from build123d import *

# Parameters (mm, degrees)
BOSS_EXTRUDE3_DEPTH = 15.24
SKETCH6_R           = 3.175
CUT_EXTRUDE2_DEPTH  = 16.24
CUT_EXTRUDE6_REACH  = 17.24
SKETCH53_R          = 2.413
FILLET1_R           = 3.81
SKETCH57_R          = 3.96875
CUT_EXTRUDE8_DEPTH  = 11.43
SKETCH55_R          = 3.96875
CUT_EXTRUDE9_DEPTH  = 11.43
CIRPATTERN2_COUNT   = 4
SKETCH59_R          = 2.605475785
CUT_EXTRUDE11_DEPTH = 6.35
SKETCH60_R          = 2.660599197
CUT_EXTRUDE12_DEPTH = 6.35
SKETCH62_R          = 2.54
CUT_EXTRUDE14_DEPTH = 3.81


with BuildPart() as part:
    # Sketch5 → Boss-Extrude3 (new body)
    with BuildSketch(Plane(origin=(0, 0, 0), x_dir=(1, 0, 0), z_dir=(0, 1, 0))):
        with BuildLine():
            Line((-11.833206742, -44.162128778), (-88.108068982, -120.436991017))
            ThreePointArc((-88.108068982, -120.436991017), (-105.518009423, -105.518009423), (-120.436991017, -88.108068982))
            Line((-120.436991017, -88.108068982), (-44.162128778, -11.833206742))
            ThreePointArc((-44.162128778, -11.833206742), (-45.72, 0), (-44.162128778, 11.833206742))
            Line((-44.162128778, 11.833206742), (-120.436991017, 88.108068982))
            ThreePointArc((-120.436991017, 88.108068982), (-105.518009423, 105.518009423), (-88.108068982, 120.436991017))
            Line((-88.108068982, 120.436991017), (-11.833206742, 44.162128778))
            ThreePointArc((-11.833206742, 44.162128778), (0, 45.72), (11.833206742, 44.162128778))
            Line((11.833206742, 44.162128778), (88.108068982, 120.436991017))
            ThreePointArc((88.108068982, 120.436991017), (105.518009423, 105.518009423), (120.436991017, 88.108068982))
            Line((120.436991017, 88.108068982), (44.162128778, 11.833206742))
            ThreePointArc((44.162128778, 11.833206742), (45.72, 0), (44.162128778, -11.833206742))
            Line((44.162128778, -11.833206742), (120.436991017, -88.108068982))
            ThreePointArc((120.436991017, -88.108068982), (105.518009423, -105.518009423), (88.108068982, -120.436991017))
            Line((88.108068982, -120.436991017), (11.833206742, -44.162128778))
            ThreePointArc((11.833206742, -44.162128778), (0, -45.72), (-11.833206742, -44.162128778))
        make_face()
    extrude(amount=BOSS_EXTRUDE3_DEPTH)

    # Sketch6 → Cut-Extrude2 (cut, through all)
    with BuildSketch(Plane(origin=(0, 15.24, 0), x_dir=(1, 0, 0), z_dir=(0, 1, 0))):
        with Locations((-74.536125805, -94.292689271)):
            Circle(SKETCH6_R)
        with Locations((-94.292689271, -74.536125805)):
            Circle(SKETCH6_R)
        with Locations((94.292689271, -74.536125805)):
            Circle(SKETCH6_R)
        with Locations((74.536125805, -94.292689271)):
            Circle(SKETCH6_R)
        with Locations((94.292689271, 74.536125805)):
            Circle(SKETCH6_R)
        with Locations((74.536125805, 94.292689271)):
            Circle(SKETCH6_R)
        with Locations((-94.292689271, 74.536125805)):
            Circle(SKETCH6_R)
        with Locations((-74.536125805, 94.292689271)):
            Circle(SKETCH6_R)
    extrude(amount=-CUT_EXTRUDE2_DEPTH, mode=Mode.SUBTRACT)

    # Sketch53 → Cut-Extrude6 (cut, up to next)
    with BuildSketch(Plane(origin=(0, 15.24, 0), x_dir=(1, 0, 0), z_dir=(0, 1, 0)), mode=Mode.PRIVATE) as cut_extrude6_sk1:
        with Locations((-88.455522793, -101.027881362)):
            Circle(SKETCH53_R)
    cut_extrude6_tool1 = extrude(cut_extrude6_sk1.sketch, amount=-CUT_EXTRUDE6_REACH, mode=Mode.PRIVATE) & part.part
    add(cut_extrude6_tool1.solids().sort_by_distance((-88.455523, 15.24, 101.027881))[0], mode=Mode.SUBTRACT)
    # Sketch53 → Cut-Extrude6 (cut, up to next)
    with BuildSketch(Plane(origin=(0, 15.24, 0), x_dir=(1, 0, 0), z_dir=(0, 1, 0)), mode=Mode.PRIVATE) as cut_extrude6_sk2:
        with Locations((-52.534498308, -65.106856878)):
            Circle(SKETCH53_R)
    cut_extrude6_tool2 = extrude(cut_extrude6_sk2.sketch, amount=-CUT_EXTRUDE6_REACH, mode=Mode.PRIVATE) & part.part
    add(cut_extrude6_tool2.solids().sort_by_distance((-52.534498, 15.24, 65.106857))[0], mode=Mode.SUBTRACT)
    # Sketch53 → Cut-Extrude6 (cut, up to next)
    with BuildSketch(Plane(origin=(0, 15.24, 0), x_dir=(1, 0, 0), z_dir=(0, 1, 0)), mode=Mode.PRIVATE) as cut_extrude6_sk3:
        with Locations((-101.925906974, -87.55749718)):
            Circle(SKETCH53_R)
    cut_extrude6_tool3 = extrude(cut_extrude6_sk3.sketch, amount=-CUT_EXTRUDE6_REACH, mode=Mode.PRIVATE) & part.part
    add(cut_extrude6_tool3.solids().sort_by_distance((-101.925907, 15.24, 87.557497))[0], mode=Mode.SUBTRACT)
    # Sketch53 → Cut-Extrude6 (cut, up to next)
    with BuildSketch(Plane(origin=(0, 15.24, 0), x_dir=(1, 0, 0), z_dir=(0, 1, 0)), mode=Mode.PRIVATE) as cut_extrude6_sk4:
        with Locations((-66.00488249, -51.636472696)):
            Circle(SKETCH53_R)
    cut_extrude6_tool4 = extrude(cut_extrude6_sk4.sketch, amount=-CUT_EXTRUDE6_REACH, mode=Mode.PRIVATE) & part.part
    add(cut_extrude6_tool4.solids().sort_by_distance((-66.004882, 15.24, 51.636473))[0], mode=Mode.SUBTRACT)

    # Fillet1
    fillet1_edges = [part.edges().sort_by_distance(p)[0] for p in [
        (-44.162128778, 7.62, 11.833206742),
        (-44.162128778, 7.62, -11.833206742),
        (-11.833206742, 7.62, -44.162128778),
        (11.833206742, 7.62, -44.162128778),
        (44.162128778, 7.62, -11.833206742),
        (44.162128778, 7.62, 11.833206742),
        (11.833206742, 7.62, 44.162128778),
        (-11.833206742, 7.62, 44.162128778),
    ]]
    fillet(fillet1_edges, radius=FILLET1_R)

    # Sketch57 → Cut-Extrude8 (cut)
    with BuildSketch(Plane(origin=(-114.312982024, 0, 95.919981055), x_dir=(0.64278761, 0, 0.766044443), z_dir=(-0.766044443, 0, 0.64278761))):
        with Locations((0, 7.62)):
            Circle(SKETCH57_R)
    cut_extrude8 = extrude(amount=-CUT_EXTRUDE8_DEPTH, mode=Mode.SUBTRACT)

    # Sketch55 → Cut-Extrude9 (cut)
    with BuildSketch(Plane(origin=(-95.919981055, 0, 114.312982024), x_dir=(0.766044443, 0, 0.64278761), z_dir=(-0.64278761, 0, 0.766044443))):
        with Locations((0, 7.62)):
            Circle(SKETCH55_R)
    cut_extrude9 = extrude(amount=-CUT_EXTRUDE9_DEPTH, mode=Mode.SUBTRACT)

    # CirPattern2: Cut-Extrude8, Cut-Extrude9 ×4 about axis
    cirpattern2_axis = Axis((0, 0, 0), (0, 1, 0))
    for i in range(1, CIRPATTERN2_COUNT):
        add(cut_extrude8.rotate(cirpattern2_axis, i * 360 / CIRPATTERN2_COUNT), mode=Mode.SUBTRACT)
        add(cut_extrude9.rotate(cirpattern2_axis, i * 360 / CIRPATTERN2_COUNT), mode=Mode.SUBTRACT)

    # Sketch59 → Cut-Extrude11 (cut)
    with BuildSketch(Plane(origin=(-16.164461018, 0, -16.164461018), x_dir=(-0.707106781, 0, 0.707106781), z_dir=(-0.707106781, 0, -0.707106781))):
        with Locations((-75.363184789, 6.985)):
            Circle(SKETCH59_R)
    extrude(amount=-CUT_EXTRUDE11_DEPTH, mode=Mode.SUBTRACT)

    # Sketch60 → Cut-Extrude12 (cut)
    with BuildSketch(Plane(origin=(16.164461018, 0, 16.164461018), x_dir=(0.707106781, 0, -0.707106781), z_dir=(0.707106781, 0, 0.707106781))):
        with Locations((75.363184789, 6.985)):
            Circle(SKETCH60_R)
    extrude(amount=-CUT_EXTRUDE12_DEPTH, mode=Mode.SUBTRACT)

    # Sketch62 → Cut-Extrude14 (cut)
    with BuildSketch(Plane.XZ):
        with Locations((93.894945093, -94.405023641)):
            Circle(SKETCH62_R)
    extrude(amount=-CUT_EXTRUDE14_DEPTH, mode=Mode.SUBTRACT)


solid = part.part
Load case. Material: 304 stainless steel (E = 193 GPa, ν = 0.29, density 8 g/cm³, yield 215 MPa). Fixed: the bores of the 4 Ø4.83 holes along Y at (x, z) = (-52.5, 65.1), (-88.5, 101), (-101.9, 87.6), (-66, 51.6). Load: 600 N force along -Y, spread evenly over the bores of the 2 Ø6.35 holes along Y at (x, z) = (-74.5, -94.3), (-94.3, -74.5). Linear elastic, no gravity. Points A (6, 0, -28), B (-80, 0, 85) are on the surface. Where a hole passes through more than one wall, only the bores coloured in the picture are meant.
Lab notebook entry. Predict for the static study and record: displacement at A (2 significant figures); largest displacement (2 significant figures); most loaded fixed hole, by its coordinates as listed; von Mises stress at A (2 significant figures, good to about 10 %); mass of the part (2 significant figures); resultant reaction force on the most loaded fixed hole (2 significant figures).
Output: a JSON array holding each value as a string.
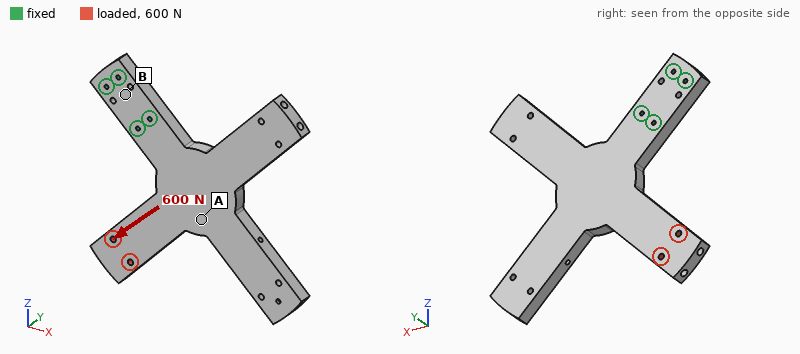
["0.082 mm", "0.37 mm", "(-66, 51.6)", "12 MPa", "3.1 kg", "2.5 kN"]
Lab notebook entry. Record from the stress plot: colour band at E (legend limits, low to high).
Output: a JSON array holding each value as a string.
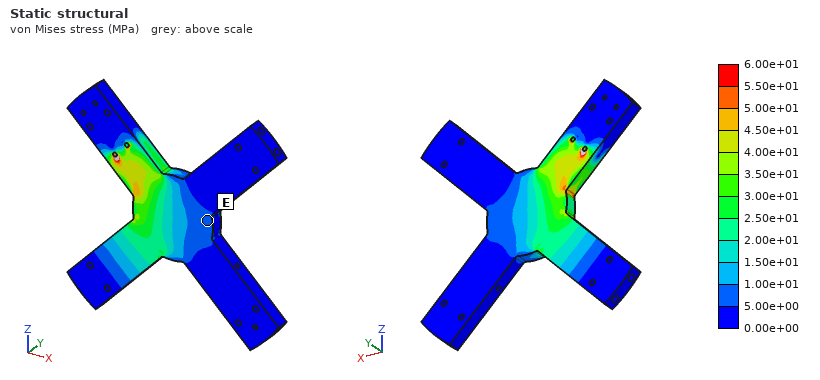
["5.00e+00 to 1.00e+01 MPa"]
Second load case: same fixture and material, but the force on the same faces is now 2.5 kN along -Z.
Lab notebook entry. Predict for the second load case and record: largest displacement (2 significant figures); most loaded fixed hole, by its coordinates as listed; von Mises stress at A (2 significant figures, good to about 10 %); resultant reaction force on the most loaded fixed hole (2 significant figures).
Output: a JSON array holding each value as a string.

["85 µm", "(-66, 51.6)", "6.4 MPa", "3.0 kN"]
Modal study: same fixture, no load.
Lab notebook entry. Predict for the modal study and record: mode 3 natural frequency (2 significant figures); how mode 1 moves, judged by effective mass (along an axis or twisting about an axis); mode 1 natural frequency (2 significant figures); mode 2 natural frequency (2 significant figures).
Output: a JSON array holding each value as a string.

["500 Hz", "along Y", "220 Hz", "320 Hz"]
